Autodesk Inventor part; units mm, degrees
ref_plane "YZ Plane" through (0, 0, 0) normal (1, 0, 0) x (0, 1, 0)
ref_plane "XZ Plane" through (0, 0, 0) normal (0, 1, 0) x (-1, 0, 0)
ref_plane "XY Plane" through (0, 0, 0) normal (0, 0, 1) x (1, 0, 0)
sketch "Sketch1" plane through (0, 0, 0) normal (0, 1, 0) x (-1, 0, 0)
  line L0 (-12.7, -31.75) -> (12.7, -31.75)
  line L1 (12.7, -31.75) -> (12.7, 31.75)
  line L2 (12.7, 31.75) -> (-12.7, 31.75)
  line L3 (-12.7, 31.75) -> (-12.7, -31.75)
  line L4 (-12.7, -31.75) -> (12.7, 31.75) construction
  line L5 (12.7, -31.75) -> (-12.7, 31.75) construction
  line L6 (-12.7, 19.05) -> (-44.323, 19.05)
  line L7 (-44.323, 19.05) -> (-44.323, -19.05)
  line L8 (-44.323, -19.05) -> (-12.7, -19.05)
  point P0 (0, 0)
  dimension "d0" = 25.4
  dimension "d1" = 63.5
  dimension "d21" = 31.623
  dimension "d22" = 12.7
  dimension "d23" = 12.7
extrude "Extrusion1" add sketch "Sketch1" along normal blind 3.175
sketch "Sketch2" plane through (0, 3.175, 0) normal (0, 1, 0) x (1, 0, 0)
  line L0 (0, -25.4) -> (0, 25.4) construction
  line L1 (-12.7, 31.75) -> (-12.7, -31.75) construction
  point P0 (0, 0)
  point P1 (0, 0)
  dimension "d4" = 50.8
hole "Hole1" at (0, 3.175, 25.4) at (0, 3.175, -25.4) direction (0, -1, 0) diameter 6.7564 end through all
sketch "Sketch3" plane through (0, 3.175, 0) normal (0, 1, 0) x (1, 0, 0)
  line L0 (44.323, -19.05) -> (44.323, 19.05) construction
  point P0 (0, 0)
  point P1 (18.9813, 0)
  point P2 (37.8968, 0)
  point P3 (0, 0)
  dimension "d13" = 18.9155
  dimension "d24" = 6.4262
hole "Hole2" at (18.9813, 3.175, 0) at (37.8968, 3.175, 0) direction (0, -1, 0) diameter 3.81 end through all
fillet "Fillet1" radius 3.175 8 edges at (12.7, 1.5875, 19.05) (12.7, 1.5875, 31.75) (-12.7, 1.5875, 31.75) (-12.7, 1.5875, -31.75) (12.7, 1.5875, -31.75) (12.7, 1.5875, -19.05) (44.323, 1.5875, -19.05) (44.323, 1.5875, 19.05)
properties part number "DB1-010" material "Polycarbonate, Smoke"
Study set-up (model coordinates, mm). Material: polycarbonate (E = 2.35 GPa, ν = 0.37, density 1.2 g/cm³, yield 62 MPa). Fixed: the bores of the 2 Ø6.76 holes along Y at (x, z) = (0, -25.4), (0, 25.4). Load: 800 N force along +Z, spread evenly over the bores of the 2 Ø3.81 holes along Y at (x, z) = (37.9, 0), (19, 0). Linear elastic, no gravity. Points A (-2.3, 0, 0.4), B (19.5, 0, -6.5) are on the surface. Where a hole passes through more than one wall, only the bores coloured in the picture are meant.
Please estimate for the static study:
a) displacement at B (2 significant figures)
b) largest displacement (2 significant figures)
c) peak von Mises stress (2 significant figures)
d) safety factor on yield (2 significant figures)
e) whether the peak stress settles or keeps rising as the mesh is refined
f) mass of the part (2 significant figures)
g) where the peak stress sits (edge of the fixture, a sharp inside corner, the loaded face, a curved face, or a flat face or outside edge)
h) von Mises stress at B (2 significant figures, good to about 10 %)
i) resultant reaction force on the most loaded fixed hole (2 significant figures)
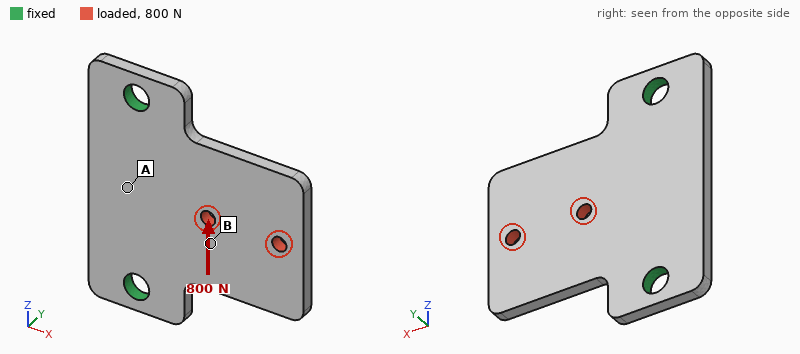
0.17 mm
0.43 mm
45 MPa
1.4
settles
10 g
a curved face
12 MPa
600 N
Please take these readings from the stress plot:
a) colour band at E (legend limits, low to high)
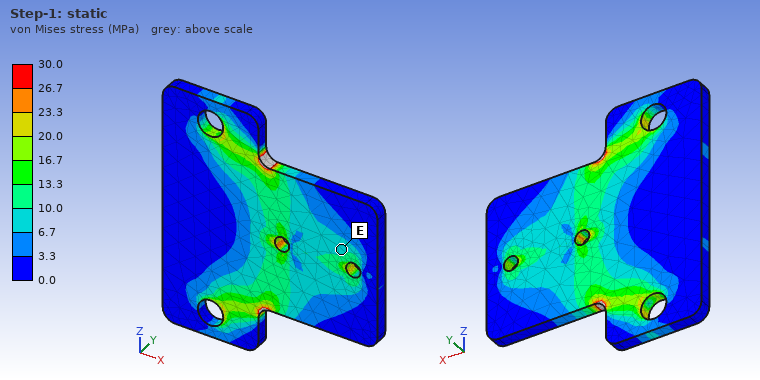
6.7 to 10.0 MPa
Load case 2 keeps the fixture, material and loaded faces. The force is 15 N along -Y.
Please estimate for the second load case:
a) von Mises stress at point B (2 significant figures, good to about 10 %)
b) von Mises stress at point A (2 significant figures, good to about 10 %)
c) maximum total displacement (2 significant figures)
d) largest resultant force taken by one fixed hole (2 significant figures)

2.6 MPa
1.3 MPa
1.00 mm
7.5 N
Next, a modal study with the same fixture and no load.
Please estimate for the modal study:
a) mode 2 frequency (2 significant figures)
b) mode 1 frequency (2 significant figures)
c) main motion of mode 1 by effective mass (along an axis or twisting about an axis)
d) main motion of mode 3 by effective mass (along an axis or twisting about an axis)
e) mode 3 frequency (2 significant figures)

1100 Hz
370 Hz
along Y
along Y
1800 Hz
